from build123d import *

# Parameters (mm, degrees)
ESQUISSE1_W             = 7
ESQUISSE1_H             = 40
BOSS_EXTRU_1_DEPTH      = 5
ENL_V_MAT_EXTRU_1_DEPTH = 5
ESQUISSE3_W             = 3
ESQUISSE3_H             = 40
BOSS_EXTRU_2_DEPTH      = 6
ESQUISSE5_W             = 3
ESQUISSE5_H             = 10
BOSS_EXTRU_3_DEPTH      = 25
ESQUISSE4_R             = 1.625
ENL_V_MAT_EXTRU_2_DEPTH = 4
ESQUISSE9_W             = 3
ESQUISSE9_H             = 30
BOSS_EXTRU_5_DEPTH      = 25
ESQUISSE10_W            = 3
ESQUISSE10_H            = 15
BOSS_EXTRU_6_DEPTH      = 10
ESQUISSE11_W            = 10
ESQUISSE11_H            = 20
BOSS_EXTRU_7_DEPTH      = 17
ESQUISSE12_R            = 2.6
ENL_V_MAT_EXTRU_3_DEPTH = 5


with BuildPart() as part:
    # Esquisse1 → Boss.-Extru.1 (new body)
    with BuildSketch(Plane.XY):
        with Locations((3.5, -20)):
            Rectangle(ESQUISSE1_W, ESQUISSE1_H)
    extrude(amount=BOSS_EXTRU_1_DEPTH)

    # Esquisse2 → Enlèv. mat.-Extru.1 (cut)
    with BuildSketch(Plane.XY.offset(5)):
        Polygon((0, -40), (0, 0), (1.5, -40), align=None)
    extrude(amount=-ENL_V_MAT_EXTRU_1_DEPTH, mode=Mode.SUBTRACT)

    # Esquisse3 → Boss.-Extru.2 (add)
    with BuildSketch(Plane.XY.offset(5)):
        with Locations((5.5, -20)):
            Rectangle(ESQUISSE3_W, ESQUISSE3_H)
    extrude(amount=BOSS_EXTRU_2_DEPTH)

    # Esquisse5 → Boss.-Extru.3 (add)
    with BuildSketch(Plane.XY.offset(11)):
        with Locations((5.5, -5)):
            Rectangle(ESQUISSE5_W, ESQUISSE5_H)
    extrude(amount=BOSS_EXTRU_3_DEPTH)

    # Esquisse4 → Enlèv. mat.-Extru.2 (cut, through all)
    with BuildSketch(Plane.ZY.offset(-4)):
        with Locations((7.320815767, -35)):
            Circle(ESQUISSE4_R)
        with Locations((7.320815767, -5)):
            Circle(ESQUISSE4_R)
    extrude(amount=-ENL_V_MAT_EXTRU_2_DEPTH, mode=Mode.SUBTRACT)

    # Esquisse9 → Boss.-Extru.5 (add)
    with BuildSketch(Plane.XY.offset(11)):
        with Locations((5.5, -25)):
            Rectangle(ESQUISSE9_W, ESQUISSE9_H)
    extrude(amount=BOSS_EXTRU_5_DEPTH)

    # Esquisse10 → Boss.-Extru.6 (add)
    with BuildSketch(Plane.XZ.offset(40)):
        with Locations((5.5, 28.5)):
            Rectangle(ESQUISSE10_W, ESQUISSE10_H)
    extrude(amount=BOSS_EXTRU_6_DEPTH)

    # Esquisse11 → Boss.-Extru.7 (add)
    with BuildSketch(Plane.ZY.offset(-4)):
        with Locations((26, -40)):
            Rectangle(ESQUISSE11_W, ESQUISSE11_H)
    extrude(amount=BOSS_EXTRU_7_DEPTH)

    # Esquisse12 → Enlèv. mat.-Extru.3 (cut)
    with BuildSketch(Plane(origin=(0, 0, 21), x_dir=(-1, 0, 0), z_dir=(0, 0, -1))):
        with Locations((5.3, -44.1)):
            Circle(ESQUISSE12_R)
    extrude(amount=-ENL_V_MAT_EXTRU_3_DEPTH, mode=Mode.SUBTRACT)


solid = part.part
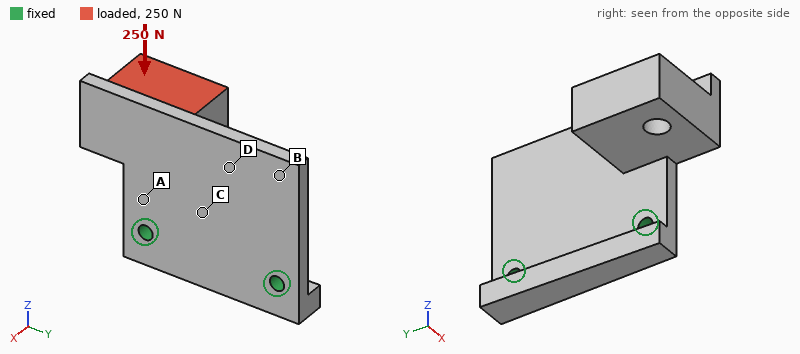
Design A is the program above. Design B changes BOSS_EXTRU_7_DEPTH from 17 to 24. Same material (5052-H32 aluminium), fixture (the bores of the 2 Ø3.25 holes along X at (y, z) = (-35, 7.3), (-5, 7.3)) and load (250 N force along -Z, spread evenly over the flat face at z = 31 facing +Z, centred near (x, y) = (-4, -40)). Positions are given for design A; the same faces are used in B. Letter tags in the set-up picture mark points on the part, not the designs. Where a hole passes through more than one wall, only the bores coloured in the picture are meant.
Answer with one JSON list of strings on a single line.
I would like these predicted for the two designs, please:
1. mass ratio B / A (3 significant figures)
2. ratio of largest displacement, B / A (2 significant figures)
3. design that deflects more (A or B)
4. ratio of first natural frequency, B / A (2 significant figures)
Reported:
["1.16", "1.6", "B", "0.78"]
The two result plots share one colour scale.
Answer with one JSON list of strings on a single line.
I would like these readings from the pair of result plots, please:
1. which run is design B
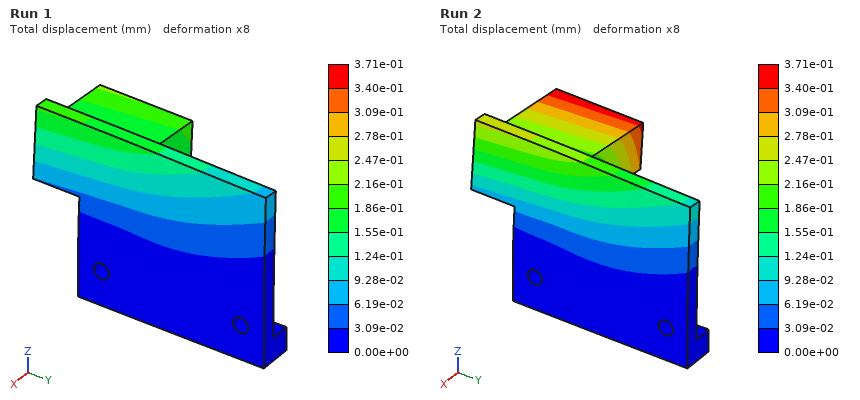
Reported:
["Run 2"]
